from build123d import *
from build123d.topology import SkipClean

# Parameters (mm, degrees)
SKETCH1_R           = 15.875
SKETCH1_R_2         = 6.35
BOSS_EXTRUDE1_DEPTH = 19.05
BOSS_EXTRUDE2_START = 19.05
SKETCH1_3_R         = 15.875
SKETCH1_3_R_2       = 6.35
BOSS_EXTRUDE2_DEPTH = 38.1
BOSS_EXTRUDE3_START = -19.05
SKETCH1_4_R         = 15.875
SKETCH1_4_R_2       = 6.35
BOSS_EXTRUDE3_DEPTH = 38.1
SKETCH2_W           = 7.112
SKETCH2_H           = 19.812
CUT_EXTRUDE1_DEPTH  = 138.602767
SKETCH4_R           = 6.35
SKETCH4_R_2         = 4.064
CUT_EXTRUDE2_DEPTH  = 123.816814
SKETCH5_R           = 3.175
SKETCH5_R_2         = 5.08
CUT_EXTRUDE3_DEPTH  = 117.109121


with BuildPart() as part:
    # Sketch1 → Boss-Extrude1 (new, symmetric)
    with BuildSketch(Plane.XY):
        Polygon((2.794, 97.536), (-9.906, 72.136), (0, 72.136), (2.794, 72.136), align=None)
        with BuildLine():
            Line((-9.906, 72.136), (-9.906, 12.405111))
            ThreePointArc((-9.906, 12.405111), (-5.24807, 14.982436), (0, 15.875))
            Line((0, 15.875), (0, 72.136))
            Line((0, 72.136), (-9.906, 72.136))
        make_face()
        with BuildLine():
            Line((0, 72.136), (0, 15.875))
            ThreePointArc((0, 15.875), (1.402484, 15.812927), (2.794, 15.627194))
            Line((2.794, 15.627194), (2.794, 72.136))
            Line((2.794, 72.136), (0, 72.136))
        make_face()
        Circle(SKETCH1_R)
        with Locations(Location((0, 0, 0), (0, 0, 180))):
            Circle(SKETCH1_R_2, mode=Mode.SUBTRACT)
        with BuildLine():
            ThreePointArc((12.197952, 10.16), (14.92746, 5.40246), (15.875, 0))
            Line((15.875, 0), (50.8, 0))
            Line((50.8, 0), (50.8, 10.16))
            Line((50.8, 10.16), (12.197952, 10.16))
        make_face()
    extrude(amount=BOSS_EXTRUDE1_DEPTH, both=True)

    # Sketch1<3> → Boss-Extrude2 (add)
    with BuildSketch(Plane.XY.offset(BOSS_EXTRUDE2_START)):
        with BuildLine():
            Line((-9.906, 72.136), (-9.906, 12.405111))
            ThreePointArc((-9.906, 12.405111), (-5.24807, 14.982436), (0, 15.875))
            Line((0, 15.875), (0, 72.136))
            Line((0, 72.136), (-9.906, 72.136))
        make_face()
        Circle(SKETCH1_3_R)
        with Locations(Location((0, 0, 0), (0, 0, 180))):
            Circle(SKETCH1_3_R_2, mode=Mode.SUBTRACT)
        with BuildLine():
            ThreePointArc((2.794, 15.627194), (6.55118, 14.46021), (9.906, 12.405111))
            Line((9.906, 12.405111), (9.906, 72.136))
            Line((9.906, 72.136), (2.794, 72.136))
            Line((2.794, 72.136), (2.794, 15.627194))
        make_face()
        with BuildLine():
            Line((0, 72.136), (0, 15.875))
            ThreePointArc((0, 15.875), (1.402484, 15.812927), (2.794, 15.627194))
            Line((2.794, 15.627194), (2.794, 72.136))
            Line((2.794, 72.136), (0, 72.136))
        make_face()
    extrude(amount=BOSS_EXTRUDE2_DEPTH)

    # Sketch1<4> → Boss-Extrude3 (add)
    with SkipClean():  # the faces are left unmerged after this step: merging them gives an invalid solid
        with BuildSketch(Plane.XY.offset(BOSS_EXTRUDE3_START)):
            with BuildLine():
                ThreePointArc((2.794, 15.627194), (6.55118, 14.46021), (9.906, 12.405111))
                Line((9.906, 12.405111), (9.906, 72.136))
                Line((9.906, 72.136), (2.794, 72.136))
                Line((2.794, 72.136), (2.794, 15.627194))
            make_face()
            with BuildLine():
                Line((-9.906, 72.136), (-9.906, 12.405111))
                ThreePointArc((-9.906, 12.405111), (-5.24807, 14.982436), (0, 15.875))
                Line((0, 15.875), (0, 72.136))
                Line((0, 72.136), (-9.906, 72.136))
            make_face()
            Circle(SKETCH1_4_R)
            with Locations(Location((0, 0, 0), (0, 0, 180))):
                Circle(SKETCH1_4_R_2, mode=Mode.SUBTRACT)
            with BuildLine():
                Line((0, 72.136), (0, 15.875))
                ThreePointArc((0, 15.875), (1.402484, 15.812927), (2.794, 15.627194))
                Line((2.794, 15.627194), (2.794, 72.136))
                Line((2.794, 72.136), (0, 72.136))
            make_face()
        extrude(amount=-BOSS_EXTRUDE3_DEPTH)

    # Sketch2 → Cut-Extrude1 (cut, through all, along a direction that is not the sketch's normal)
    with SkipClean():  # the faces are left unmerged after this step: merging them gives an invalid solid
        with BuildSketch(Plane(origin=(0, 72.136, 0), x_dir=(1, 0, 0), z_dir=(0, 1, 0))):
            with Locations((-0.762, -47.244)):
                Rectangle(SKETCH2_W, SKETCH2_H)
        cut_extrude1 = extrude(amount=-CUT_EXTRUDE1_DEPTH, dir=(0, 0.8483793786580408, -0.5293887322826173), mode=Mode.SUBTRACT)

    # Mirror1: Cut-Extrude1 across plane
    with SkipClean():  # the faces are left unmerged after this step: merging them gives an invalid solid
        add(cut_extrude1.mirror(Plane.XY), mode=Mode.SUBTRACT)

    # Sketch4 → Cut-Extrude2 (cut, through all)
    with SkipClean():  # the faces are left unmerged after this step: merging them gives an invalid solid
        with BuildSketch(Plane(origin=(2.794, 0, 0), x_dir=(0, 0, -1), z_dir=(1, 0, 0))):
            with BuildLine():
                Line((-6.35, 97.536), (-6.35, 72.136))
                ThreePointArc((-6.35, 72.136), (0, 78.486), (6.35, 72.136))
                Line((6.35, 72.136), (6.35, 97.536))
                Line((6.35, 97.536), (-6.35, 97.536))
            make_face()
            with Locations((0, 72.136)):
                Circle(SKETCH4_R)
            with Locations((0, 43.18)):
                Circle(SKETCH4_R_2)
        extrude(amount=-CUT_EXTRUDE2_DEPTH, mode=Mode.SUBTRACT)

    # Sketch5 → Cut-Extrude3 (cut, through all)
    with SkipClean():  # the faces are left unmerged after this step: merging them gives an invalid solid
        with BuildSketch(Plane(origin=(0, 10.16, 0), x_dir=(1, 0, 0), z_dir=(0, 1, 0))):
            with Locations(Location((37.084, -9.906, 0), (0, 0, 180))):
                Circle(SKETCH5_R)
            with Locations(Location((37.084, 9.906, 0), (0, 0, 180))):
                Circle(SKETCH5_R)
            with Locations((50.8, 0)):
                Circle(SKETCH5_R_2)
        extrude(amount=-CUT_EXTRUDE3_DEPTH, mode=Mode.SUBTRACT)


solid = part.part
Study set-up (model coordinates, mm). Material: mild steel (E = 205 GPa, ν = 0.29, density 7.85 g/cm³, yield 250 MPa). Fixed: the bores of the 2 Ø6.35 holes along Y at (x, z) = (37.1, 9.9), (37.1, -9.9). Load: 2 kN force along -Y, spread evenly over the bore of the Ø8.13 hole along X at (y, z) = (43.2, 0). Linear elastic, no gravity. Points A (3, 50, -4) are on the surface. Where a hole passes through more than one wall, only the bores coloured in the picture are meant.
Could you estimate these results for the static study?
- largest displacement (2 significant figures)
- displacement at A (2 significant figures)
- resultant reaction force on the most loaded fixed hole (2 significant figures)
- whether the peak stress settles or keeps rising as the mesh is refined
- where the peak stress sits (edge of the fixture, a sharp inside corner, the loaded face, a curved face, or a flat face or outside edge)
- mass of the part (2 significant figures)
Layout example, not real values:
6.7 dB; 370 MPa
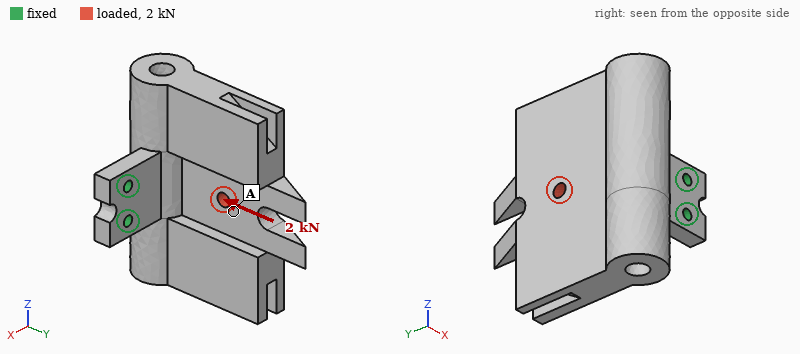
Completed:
0.19 mm; 0.10 mm; 1.0 kN; keeps rising; edge of the fixture; 1.6 kg
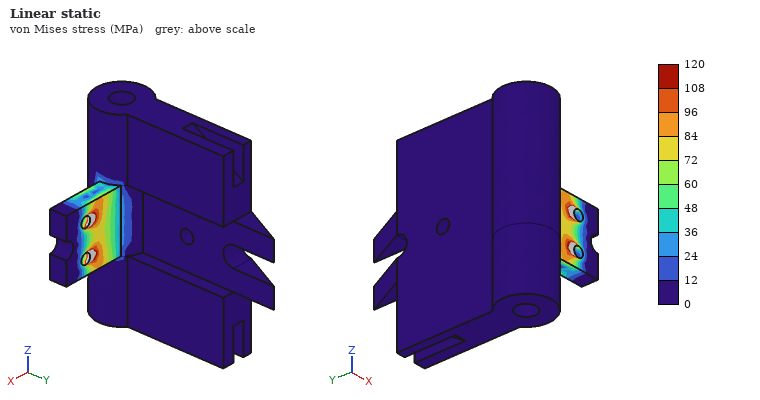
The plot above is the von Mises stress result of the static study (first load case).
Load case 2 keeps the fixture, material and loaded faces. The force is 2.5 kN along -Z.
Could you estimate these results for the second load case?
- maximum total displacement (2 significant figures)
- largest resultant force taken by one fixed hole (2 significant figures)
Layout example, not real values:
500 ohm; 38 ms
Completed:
0.14 mm; 5.4 kN
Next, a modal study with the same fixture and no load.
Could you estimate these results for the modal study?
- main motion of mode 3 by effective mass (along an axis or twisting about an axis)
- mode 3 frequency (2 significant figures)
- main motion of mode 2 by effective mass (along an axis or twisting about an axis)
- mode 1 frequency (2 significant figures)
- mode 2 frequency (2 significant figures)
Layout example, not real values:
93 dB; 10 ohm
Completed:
along Z; 1600 Hz; along Z; 510 Hz; 710 Hz
